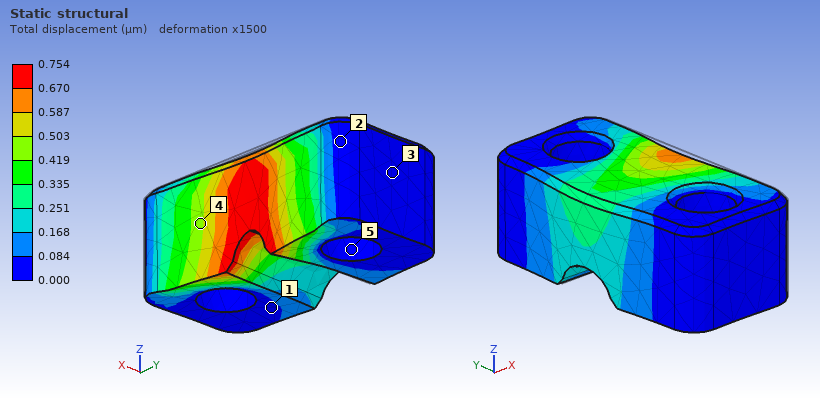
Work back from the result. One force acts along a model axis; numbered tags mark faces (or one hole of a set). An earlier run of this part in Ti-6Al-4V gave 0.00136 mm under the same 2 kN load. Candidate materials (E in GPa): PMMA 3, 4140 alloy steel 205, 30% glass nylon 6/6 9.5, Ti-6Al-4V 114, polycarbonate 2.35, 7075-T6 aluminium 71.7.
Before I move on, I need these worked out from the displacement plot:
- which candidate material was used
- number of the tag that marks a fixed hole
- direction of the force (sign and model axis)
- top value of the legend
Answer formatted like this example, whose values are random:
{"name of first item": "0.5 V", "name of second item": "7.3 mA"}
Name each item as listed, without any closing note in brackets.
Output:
{"which candidate material was used": "4140 alloy steel", "number of the tag that marks a fixed hole": "5", "direction of the force": "-X", "top value of the legend": "0.754 µm"}
